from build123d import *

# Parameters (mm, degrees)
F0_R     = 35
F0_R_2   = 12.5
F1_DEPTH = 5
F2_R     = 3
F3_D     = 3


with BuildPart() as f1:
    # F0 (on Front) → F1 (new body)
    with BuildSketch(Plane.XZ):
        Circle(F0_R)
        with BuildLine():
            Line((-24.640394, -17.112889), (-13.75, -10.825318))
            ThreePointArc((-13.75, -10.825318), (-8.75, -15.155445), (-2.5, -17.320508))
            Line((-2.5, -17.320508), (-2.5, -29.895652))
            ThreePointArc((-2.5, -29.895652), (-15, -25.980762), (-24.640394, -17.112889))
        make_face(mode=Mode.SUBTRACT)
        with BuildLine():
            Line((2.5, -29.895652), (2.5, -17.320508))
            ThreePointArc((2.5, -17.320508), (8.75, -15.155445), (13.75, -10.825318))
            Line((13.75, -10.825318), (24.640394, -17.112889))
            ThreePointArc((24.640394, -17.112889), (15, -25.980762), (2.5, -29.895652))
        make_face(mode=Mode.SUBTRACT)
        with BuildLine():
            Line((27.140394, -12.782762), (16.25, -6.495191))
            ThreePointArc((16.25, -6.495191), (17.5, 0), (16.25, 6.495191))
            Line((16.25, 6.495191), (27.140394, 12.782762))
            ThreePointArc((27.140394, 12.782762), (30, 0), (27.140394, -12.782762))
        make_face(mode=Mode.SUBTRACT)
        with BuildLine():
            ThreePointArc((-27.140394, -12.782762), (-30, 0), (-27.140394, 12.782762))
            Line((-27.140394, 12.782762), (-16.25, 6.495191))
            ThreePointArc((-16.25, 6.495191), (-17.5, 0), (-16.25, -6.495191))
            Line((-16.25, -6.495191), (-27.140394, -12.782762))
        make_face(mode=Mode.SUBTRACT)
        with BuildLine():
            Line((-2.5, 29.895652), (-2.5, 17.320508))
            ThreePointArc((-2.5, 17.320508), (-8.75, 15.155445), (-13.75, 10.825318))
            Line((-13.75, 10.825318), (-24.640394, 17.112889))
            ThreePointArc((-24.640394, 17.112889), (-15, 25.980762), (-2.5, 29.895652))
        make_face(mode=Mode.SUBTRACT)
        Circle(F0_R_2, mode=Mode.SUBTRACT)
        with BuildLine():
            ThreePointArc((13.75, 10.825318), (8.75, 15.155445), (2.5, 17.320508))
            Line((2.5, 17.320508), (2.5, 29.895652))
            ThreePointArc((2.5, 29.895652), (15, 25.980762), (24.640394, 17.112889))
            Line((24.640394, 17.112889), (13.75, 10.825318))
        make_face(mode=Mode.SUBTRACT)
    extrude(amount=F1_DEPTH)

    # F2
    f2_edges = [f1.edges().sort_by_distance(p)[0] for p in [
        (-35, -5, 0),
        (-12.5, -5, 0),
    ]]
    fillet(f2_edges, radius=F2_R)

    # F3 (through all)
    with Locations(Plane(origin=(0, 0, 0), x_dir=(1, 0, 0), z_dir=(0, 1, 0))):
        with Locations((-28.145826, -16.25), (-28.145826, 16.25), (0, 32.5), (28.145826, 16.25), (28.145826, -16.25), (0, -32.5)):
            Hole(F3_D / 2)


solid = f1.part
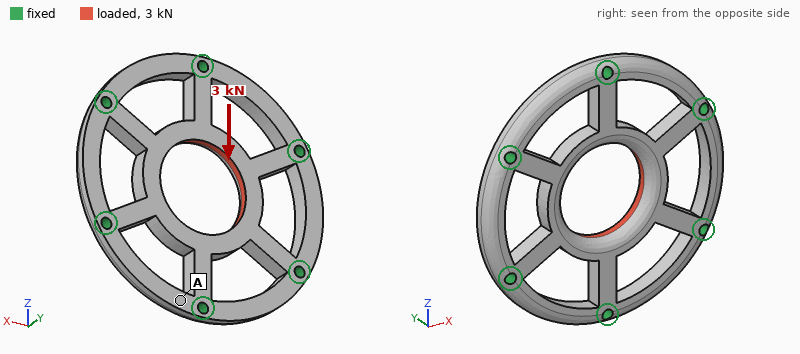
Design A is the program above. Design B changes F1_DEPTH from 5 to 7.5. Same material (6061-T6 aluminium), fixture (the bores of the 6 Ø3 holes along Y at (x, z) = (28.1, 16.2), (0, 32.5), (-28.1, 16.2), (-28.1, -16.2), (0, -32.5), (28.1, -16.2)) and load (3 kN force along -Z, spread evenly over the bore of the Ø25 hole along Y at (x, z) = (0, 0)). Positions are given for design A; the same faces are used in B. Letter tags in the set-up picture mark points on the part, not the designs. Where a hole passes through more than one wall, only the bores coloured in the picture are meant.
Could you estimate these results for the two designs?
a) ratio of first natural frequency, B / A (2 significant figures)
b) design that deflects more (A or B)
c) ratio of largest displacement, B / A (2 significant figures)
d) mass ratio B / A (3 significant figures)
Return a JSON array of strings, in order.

["1.4", "A", "0.63", "1.53"]
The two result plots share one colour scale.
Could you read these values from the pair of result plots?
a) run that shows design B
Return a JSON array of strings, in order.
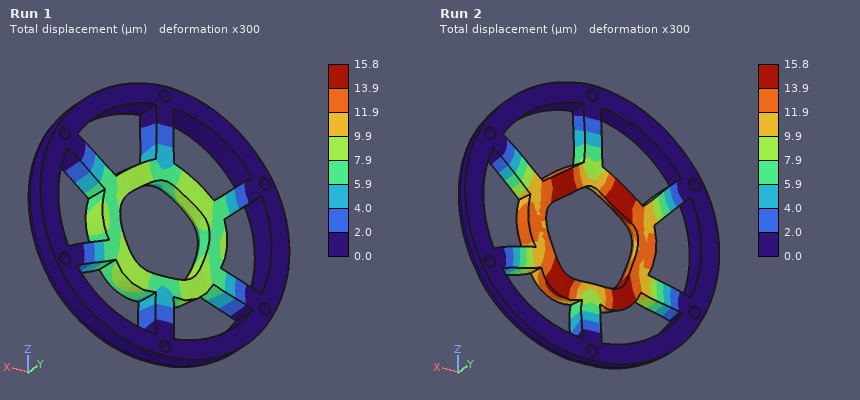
["Run 1"]
